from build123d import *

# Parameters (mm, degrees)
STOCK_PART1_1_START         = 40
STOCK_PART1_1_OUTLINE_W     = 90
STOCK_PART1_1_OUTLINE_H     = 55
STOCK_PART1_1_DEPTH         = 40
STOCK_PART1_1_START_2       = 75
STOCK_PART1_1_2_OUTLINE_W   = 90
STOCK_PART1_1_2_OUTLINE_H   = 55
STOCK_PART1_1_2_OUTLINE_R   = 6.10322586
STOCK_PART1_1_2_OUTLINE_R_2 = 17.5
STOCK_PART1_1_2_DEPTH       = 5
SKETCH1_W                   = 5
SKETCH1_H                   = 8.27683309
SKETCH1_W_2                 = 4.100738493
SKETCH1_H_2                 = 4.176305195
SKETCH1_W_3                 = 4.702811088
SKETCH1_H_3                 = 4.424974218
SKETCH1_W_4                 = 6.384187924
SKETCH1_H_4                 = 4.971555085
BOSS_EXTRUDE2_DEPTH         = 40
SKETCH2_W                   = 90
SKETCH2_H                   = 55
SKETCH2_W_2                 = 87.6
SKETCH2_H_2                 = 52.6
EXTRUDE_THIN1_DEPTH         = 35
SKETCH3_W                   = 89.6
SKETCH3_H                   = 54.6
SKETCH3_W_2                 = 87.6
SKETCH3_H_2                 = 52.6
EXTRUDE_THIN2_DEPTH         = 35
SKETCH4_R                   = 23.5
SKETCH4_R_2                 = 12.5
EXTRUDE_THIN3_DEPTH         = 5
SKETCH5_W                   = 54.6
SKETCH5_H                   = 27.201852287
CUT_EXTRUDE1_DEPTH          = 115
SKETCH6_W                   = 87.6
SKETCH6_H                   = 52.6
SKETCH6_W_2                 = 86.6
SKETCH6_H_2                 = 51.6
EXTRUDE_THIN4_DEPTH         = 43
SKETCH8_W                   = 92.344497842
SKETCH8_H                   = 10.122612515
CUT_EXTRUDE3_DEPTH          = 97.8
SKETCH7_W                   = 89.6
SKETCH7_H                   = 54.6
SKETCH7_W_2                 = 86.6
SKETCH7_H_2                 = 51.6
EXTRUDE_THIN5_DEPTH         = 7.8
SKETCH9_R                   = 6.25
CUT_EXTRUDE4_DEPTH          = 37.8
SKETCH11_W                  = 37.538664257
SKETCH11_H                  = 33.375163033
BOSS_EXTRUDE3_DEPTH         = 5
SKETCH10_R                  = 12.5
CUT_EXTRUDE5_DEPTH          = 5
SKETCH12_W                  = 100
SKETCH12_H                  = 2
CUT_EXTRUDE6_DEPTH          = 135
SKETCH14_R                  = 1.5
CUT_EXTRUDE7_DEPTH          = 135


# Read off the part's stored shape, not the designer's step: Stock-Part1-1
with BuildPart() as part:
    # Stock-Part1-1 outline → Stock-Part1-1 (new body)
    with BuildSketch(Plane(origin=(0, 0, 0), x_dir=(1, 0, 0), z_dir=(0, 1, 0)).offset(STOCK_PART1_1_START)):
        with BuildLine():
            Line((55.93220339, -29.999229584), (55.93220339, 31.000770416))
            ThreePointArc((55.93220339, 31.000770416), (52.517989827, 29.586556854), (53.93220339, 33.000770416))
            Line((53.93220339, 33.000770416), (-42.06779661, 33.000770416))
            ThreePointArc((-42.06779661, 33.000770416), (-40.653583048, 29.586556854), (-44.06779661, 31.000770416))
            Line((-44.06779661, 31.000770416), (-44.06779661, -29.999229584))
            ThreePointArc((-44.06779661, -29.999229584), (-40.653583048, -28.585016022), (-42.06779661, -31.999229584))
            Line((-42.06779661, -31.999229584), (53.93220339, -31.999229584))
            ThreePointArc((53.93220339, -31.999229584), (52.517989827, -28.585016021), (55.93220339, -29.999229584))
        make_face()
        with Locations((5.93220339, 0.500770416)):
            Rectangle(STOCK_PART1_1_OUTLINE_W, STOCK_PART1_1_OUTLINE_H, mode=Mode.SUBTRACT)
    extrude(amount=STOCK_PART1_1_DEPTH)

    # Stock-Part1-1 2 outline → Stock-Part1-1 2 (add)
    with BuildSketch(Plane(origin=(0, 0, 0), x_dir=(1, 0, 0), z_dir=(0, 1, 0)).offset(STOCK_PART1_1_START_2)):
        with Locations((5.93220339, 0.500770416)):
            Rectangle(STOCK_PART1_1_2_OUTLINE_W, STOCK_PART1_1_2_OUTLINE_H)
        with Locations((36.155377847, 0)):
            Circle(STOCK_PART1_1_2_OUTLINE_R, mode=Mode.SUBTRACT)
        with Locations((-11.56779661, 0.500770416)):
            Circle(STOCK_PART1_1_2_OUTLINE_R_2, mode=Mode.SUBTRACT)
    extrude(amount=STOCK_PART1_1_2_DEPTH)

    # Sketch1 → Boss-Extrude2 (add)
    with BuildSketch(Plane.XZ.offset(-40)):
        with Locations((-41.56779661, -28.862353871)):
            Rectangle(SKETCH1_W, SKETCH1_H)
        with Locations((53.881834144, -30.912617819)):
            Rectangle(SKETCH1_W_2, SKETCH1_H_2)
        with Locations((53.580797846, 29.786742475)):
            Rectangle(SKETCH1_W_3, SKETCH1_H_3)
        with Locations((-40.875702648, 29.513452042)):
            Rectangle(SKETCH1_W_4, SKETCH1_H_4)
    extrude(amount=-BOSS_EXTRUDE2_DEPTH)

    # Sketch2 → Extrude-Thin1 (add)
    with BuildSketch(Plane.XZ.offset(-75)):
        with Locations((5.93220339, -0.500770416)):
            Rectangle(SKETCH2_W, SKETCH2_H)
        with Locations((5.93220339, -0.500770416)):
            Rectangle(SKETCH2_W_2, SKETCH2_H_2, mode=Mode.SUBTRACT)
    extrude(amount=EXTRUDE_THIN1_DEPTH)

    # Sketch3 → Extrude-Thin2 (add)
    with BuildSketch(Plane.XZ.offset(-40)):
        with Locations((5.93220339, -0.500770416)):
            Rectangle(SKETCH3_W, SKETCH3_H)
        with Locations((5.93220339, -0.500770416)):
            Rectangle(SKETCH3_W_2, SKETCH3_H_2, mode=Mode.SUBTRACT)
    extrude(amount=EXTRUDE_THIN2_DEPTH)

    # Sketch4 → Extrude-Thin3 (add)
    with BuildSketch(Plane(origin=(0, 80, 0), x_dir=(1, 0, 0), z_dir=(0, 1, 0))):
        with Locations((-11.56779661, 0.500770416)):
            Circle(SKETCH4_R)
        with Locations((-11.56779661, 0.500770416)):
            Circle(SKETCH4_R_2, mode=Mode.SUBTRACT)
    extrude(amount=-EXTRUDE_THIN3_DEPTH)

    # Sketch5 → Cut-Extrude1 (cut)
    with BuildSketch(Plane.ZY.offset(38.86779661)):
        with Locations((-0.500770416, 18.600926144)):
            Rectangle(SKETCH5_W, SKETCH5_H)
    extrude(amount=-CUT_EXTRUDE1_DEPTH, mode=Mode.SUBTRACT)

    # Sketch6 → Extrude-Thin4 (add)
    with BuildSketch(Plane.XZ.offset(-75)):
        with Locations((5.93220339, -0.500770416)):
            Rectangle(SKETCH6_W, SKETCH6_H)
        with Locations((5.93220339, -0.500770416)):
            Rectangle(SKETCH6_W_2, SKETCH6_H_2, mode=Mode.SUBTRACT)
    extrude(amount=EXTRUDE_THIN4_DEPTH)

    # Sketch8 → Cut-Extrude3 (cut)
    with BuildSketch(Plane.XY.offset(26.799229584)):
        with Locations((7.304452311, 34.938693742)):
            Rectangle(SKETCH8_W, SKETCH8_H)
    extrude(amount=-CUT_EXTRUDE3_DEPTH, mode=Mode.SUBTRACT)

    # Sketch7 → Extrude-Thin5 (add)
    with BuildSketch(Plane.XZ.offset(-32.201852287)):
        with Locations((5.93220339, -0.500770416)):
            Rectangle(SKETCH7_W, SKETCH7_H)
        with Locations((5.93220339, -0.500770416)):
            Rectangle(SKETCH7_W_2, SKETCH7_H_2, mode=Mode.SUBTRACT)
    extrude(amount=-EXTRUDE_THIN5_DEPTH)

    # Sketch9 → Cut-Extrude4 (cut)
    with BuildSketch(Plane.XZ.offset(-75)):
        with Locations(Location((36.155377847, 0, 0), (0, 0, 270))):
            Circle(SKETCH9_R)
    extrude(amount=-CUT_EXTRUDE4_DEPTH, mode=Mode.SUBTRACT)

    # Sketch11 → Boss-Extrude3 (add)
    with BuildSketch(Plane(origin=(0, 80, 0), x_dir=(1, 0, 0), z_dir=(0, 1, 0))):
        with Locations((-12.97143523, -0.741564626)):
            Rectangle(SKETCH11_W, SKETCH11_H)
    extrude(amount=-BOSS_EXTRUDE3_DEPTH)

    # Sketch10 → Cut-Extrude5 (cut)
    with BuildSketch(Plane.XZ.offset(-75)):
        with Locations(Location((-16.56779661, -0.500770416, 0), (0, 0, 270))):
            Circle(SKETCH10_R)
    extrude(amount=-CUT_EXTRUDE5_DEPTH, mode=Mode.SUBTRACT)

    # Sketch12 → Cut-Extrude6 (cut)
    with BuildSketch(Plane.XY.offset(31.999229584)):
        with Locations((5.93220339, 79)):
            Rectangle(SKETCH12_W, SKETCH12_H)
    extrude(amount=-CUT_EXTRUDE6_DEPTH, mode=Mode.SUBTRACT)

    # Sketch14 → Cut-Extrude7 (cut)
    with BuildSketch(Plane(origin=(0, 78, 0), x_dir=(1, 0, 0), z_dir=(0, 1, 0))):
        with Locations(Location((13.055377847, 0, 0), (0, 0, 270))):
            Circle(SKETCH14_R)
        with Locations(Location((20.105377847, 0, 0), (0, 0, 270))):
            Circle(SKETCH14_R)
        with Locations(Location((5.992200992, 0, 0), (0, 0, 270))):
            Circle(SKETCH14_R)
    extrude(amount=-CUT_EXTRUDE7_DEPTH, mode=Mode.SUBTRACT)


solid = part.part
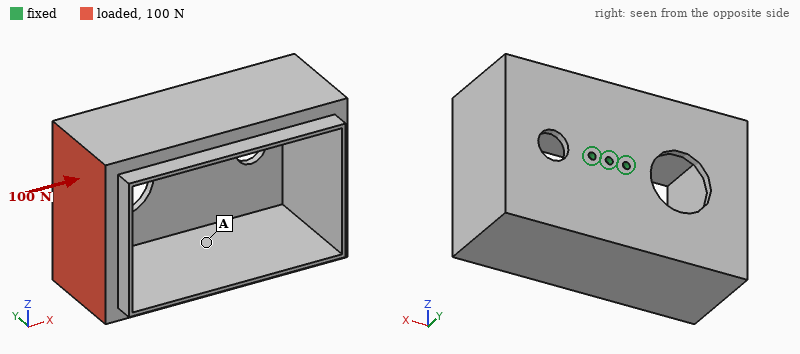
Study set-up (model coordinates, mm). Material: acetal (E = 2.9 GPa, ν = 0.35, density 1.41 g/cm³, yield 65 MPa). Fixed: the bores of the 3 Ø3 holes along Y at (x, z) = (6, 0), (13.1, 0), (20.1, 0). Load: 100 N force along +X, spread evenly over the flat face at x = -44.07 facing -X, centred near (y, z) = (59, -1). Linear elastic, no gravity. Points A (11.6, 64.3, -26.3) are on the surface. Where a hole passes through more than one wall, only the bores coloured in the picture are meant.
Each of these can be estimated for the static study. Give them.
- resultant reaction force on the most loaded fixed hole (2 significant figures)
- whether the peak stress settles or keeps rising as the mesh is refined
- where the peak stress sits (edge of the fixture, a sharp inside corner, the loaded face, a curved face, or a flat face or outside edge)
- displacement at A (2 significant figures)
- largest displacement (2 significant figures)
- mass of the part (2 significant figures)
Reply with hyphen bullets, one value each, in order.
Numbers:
- 93 N
- keeps rising
- edge of the fixture
- 0.26 mm
- 1.4 mm
- 130 g
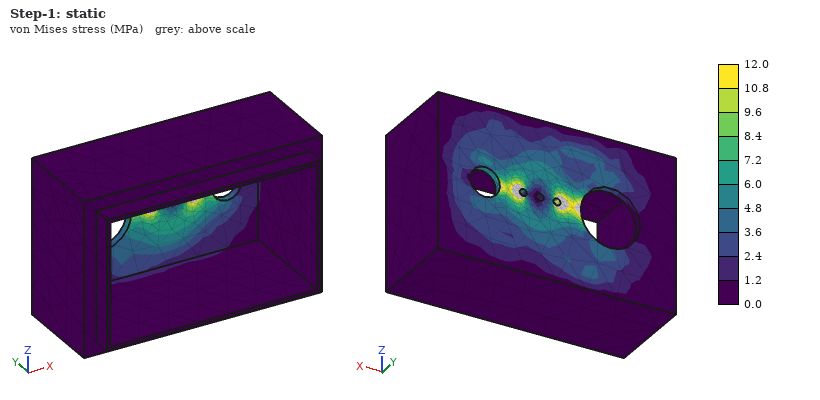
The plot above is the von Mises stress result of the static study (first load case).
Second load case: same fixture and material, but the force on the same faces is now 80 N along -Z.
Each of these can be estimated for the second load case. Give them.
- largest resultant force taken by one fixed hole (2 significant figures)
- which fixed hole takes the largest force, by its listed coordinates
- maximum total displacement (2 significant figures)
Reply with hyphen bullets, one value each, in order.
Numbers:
- 310 N
- (6, 0)
- 1.4 mm
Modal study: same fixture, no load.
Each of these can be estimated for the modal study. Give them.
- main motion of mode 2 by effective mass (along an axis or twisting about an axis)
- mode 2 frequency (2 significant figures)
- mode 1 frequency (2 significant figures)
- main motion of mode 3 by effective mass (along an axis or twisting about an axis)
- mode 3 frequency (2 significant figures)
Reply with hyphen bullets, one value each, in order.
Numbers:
- along Z
- 110 Hz
- 100 Hz
- along Y
- 300 Hz
